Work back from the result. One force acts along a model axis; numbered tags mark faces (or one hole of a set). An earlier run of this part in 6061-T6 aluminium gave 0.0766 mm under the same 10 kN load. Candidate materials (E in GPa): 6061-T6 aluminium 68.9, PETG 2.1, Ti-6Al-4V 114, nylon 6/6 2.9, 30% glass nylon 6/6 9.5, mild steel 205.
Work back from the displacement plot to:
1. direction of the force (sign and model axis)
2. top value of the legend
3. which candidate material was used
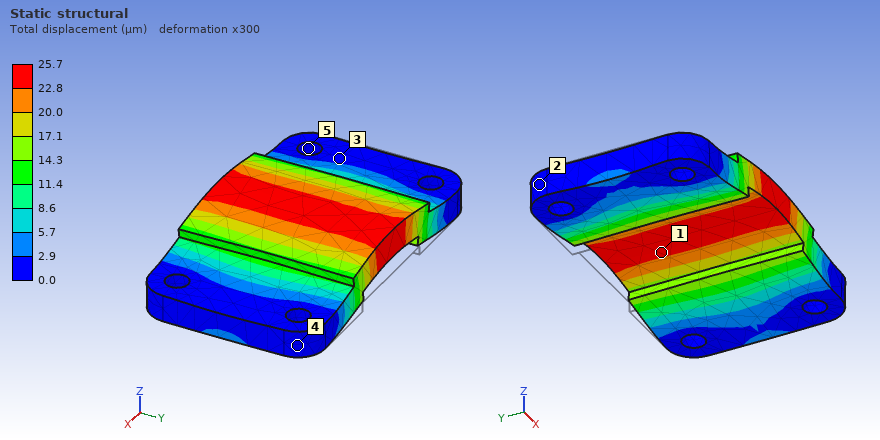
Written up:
+Z
25.7 µm
mild steel
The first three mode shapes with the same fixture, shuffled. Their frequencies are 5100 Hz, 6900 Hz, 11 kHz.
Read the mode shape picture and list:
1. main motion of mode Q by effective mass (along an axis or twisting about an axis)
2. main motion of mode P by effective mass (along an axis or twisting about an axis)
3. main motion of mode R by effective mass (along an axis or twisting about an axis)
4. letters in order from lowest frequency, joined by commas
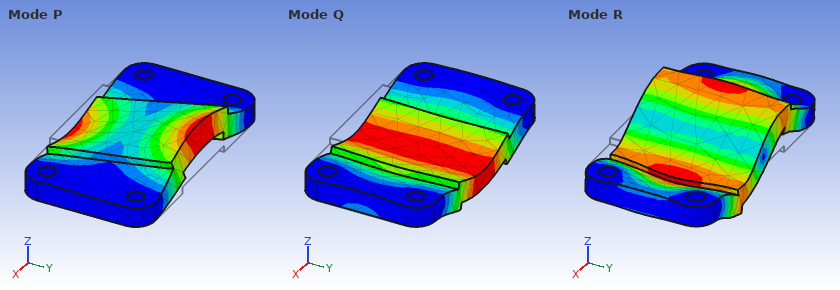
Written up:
along Z
twisting about X
twisting about Y
Q, P, R
